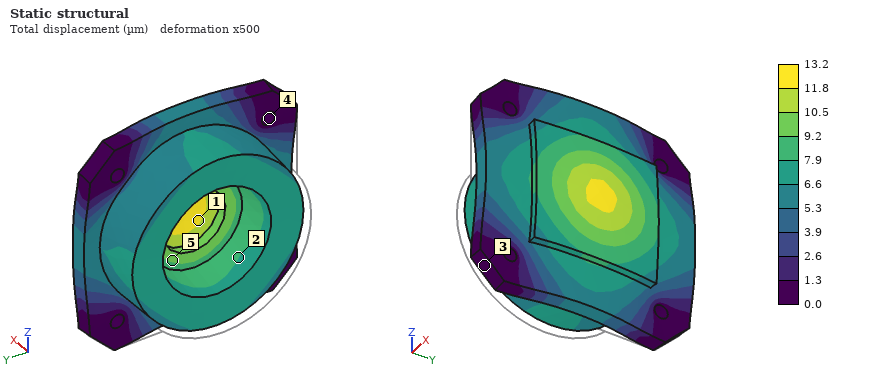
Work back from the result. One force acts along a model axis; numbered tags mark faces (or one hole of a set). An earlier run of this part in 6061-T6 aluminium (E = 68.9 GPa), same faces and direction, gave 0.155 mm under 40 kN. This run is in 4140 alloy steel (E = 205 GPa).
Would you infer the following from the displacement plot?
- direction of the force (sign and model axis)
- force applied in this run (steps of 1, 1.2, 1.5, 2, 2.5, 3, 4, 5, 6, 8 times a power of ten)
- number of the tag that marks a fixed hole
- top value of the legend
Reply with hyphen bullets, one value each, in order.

- +X
- 10 kN
- 4
- 13.2 µm
